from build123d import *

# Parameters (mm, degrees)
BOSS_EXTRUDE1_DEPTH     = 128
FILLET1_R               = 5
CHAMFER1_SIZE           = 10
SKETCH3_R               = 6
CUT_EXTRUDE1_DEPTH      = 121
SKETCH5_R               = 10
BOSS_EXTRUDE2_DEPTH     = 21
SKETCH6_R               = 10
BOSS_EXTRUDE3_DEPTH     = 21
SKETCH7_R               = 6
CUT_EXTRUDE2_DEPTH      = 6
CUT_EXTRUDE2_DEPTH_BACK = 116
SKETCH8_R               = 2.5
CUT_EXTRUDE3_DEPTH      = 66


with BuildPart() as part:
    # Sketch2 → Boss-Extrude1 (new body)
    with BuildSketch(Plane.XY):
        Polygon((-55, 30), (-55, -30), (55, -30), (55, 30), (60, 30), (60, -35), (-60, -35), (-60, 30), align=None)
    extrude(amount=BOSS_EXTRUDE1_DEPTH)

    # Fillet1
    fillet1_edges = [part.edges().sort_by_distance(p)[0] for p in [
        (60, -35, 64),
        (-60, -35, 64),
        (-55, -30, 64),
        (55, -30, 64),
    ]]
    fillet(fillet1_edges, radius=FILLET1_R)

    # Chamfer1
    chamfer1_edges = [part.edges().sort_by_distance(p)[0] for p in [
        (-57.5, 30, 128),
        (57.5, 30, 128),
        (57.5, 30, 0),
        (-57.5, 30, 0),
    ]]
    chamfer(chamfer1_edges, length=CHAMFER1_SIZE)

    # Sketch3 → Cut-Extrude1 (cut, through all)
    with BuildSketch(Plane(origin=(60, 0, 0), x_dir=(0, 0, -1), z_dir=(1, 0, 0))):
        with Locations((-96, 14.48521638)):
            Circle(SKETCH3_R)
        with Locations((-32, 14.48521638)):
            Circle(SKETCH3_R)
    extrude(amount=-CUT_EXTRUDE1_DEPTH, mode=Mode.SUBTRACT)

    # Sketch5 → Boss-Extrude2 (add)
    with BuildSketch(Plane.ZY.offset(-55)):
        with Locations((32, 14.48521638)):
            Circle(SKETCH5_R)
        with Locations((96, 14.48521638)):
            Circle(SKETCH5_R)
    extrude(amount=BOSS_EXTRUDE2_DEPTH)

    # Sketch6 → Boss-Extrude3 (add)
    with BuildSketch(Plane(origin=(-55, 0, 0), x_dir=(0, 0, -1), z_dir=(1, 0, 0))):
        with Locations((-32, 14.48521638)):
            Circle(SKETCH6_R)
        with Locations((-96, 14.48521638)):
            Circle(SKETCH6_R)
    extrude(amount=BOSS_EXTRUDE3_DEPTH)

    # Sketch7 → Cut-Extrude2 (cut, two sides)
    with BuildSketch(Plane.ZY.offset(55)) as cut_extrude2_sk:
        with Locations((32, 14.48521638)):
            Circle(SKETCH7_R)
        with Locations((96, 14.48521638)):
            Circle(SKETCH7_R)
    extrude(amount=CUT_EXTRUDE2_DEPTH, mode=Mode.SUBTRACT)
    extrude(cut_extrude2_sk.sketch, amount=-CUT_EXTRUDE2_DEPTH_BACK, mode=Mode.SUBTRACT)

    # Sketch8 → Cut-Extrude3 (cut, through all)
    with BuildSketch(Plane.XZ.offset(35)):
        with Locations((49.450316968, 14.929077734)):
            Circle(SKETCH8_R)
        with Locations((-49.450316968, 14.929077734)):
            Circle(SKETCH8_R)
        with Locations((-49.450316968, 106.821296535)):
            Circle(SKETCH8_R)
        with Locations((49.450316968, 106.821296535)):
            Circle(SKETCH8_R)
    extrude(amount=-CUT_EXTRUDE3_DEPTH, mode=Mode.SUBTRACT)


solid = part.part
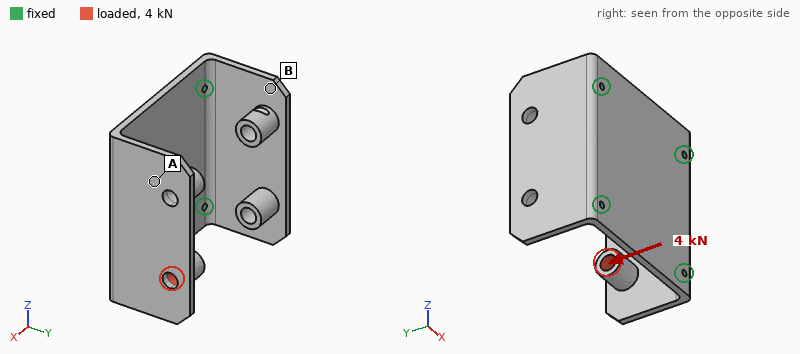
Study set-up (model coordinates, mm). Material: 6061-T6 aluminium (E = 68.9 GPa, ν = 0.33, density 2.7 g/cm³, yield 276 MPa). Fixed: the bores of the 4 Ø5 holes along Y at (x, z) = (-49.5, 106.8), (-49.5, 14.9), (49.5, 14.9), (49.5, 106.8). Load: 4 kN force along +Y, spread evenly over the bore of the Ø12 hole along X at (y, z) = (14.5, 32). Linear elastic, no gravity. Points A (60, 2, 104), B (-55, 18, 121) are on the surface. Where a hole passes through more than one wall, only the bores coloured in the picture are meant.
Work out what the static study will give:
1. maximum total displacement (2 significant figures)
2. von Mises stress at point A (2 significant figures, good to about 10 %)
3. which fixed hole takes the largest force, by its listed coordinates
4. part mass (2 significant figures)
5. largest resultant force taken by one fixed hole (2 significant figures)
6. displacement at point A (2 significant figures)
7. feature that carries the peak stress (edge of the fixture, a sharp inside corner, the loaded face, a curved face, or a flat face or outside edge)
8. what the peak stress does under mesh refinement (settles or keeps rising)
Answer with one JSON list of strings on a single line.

["1.5 mm", "45 MPa", "(49.5, 14.9)", "450 g", "3.3 kN", "0.26 mm", "edge of the fixture", "keeps rising"]
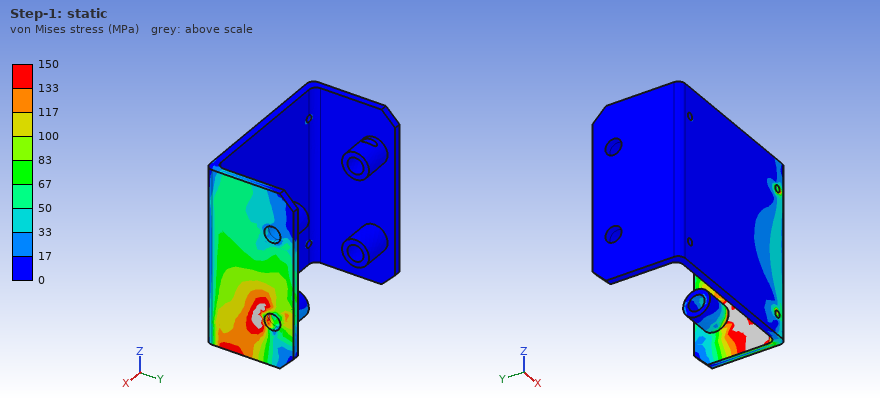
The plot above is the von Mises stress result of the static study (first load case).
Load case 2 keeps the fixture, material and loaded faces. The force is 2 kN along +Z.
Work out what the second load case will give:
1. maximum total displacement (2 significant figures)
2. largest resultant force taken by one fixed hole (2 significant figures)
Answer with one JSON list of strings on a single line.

["0.36 mm", "1.4 kN"]
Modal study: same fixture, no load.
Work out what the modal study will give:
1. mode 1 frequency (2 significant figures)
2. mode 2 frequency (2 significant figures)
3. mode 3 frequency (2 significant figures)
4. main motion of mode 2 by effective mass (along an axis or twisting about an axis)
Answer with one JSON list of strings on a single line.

["760 Hz", "790 Hz", "1400 Hz", "along X"]
